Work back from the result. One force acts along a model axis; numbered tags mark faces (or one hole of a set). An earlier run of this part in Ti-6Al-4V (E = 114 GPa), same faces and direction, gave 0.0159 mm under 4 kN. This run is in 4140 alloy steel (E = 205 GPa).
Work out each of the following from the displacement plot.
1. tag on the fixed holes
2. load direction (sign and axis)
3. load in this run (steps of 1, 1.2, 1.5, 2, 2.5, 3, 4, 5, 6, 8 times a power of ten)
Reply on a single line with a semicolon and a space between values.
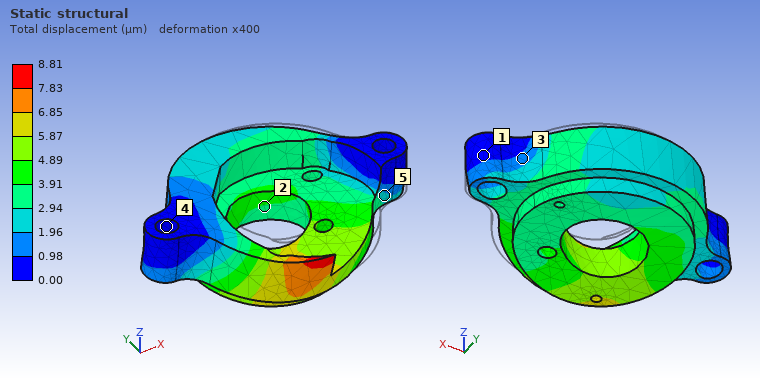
4; -X; 4 kN
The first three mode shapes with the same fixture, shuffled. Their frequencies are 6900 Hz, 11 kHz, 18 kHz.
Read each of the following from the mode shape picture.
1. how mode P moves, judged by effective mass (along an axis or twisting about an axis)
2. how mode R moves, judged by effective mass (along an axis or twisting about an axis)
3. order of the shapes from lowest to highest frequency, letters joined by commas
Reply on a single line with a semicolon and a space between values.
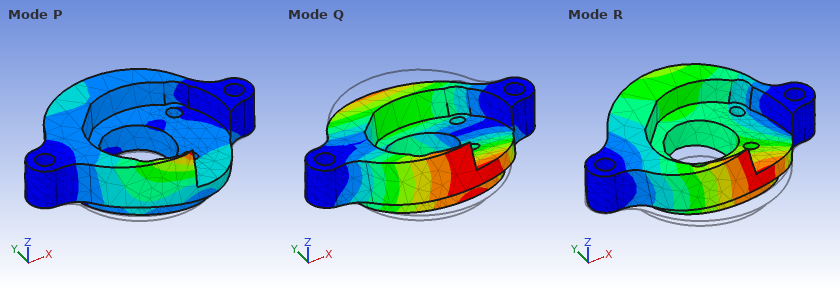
along Y; along Z; Q, R, P
